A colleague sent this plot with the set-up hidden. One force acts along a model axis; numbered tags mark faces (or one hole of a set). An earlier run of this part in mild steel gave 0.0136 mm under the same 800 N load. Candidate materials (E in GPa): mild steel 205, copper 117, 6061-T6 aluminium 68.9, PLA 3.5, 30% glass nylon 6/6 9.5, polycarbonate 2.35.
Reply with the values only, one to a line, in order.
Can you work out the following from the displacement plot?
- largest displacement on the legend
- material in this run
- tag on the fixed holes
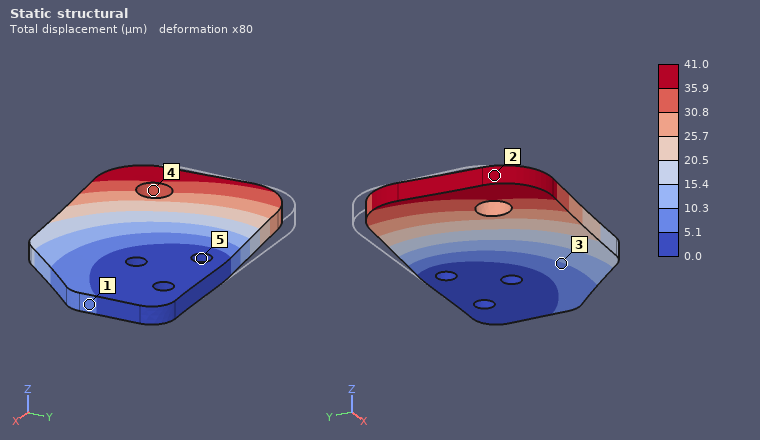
41.0 µm
6061-T6 aluminium
5
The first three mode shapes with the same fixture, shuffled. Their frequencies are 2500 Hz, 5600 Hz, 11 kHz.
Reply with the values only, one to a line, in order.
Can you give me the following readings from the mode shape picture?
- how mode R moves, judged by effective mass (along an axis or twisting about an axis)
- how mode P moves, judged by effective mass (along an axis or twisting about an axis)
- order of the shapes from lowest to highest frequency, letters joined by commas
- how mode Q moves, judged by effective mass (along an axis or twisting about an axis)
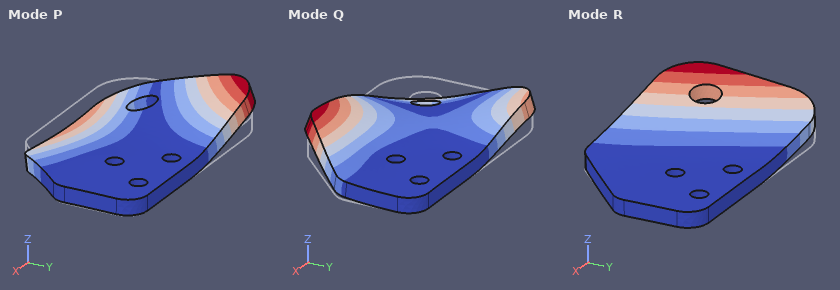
along Z
twisting about X
R, P, Q
along Z
